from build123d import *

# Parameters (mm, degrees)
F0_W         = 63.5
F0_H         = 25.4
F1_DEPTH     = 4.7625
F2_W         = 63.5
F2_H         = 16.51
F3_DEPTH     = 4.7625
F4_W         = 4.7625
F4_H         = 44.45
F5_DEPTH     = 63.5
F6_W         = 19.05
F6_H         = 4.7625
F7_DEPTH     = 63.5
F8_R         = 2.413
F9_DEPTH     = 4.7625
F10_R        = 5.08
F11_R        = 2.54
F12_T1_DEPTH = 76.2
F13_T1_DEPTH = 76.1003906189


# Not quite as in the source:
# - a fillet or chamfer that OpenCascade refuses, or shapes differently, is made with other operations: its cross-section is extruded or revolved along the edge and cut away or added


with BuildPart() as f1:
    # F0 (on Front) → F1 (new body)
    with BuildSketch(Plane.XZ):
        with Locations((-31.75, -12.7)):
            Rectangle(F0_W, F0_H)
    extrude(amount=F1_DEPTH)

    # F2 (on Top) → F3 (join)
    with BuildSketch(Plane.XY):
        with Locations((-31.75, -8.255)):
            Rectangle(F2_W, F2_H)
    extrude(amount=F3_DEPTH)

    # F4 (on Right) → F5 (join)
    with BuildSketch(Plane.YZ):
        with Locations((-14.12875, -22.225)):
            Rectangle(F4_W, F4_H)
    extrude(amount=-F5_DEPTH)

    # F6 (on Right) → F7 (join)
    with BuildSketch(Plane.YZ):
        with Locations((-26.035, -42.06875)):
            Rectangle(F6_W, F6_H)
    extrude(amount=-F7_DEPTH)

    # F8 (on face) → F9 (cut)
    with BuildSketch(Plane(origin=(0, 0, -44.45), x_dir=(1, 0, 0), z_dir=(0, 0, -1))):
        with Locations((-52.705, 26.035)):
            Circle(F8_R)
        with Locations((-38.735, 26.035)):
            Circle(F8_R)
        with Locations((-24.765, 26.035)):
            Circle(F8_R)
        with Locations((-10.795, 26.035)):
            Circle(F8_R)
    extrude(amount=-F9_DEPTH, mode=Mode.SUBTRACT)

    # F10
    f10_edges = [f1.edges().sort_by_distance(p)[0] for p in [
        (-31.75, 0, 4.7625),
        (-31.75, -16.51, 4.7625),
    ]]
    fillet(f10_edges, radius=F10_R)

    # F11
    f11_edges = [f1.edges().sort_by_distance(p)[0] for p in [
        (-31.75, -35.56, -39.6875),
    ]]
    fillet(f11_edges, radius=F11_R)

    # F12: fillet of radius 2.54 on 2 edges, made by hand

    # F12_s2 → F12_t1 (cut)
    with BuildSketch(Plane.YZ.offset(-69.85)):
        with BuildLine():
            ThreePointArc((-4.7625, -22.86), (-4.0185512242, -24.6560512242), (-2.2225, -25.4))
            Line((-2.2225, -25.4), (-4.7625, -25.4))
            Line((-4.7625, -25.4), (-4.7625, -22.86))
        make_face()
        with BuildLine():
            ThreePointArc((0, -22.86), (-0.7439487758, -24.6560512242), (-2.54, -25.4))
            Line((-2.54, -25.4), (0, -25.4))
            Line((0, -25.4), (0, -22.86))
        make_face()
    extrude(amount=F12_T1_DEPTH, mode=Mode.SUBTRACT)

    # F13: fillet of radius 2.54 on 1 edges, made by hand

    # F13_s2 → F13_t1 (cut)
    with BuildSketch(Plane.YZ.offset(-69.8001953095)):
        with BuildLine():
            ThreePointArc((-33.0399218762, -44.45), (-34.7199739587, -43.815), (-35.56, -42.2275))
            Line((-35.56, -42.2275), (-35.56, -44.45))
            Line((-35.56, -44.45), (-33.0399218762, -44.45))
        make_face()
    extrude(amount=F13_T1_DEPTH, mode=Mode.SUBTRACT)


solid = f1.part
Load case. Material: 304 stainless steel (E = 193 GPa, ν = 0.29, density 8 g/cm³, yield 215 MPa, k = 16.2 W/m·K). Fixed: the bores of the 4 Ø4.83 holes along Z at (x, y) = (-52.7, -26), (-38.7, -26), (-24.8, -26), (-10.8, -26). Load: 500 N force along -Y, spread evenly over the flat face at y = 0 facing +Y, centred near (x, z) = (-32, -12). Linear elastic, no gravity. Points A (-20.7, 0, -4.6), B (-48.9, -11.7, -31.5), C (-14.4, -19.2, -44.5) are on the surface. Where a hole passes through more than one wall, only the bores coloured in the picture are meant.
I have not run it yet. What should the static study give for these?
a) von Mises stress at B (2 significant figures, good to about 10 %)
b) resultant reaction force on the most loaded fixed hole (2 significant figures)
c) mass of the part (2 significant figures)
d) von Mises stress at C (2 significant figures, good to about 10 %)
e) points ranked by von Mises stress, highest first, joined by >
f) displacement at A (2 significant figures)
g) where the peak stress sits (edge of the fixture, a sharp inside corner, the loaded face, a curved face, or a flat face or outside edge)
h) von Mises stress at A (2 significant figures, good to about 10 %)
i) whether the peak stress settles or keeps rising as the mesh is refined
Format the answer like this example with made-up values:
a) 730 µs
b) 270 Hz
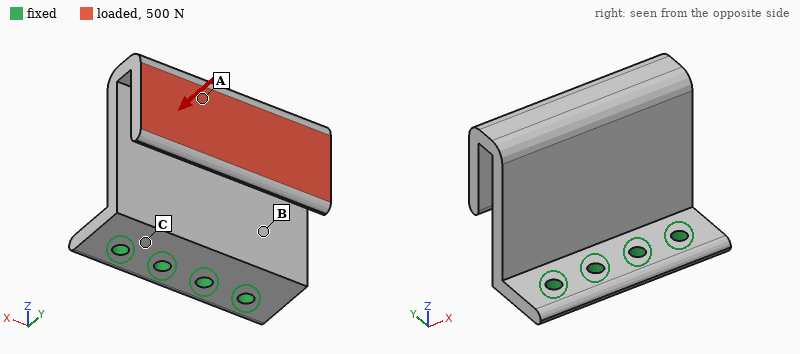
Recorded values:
a) 37 MPa
b) 140 N
c) 240 g
d) 55 MPa
e) C > B > A
f) 0.12 mm
g) edge of the fixture
h) 15 MPa
i) keeps rising
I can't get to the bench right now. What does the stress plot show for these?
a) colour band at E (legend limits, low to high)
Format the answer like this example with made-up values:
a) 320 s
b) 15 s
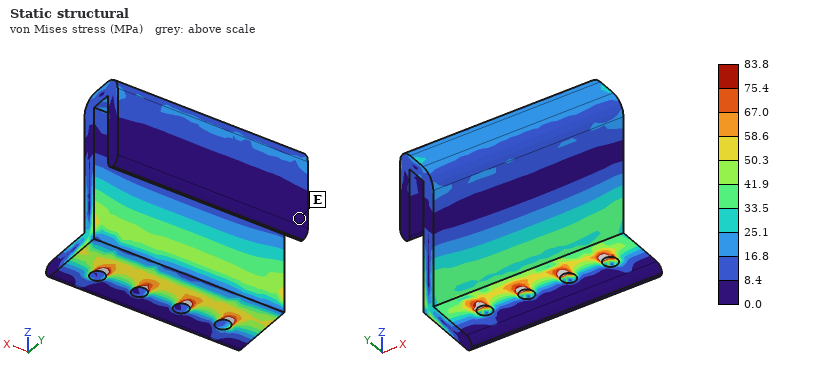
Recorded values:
a) 0.0 to 8.4 MPa
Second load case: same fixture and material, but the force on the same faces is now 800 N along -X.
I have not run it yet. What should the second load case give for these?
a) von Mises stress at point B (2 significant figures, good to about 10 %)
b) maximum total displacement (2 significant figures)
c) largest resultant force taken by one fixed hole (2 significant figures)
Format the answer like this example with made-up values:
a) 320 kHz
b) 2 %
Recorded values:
a) 29 MPa
b) 67 µm
c) 670 N
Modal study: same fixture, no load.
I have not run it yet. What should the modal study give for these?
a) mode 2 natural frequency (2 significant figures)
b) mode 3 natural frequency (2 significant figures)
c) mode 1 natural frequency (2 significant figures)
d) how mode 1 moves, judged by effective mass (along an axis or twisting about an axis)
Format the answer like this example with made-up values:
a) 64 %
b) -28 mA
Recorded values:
a) 1700 Hz
b) 2300 Hz
c) 810 Hz
d) along Y
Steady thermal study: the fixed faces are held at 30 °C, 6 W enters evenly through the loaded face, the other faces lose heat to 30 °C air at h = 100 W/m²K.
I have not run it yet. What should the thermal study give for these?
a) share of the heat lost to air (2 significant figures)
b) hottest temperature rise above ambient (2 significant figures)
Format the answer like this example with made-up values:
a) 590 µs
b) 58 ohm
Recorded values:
a) 97 %
b) 17 K
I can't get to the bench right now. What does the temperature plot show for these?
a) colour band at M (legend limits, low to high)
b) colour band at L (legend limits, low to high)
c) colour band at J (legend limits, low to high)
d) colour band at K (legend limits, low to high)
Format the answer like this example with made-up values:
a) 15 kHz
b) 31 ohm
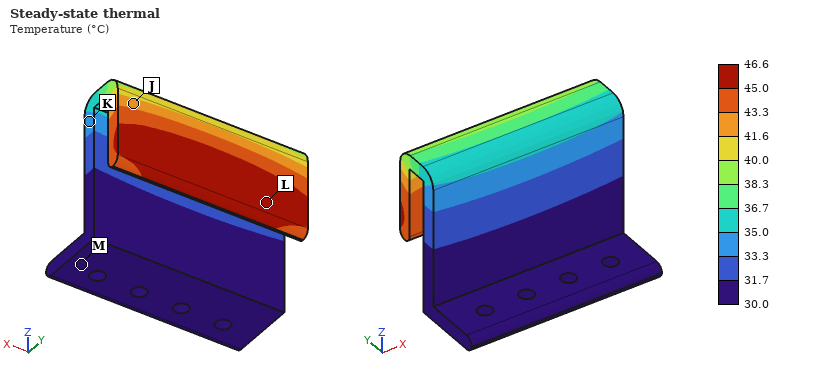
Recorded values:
a) 30.0 to 31.7 °C
b) 45.0 to 46.6 °C
c) 41.6 to 43.3 °C
d) 33.3 to 35.0 °C
